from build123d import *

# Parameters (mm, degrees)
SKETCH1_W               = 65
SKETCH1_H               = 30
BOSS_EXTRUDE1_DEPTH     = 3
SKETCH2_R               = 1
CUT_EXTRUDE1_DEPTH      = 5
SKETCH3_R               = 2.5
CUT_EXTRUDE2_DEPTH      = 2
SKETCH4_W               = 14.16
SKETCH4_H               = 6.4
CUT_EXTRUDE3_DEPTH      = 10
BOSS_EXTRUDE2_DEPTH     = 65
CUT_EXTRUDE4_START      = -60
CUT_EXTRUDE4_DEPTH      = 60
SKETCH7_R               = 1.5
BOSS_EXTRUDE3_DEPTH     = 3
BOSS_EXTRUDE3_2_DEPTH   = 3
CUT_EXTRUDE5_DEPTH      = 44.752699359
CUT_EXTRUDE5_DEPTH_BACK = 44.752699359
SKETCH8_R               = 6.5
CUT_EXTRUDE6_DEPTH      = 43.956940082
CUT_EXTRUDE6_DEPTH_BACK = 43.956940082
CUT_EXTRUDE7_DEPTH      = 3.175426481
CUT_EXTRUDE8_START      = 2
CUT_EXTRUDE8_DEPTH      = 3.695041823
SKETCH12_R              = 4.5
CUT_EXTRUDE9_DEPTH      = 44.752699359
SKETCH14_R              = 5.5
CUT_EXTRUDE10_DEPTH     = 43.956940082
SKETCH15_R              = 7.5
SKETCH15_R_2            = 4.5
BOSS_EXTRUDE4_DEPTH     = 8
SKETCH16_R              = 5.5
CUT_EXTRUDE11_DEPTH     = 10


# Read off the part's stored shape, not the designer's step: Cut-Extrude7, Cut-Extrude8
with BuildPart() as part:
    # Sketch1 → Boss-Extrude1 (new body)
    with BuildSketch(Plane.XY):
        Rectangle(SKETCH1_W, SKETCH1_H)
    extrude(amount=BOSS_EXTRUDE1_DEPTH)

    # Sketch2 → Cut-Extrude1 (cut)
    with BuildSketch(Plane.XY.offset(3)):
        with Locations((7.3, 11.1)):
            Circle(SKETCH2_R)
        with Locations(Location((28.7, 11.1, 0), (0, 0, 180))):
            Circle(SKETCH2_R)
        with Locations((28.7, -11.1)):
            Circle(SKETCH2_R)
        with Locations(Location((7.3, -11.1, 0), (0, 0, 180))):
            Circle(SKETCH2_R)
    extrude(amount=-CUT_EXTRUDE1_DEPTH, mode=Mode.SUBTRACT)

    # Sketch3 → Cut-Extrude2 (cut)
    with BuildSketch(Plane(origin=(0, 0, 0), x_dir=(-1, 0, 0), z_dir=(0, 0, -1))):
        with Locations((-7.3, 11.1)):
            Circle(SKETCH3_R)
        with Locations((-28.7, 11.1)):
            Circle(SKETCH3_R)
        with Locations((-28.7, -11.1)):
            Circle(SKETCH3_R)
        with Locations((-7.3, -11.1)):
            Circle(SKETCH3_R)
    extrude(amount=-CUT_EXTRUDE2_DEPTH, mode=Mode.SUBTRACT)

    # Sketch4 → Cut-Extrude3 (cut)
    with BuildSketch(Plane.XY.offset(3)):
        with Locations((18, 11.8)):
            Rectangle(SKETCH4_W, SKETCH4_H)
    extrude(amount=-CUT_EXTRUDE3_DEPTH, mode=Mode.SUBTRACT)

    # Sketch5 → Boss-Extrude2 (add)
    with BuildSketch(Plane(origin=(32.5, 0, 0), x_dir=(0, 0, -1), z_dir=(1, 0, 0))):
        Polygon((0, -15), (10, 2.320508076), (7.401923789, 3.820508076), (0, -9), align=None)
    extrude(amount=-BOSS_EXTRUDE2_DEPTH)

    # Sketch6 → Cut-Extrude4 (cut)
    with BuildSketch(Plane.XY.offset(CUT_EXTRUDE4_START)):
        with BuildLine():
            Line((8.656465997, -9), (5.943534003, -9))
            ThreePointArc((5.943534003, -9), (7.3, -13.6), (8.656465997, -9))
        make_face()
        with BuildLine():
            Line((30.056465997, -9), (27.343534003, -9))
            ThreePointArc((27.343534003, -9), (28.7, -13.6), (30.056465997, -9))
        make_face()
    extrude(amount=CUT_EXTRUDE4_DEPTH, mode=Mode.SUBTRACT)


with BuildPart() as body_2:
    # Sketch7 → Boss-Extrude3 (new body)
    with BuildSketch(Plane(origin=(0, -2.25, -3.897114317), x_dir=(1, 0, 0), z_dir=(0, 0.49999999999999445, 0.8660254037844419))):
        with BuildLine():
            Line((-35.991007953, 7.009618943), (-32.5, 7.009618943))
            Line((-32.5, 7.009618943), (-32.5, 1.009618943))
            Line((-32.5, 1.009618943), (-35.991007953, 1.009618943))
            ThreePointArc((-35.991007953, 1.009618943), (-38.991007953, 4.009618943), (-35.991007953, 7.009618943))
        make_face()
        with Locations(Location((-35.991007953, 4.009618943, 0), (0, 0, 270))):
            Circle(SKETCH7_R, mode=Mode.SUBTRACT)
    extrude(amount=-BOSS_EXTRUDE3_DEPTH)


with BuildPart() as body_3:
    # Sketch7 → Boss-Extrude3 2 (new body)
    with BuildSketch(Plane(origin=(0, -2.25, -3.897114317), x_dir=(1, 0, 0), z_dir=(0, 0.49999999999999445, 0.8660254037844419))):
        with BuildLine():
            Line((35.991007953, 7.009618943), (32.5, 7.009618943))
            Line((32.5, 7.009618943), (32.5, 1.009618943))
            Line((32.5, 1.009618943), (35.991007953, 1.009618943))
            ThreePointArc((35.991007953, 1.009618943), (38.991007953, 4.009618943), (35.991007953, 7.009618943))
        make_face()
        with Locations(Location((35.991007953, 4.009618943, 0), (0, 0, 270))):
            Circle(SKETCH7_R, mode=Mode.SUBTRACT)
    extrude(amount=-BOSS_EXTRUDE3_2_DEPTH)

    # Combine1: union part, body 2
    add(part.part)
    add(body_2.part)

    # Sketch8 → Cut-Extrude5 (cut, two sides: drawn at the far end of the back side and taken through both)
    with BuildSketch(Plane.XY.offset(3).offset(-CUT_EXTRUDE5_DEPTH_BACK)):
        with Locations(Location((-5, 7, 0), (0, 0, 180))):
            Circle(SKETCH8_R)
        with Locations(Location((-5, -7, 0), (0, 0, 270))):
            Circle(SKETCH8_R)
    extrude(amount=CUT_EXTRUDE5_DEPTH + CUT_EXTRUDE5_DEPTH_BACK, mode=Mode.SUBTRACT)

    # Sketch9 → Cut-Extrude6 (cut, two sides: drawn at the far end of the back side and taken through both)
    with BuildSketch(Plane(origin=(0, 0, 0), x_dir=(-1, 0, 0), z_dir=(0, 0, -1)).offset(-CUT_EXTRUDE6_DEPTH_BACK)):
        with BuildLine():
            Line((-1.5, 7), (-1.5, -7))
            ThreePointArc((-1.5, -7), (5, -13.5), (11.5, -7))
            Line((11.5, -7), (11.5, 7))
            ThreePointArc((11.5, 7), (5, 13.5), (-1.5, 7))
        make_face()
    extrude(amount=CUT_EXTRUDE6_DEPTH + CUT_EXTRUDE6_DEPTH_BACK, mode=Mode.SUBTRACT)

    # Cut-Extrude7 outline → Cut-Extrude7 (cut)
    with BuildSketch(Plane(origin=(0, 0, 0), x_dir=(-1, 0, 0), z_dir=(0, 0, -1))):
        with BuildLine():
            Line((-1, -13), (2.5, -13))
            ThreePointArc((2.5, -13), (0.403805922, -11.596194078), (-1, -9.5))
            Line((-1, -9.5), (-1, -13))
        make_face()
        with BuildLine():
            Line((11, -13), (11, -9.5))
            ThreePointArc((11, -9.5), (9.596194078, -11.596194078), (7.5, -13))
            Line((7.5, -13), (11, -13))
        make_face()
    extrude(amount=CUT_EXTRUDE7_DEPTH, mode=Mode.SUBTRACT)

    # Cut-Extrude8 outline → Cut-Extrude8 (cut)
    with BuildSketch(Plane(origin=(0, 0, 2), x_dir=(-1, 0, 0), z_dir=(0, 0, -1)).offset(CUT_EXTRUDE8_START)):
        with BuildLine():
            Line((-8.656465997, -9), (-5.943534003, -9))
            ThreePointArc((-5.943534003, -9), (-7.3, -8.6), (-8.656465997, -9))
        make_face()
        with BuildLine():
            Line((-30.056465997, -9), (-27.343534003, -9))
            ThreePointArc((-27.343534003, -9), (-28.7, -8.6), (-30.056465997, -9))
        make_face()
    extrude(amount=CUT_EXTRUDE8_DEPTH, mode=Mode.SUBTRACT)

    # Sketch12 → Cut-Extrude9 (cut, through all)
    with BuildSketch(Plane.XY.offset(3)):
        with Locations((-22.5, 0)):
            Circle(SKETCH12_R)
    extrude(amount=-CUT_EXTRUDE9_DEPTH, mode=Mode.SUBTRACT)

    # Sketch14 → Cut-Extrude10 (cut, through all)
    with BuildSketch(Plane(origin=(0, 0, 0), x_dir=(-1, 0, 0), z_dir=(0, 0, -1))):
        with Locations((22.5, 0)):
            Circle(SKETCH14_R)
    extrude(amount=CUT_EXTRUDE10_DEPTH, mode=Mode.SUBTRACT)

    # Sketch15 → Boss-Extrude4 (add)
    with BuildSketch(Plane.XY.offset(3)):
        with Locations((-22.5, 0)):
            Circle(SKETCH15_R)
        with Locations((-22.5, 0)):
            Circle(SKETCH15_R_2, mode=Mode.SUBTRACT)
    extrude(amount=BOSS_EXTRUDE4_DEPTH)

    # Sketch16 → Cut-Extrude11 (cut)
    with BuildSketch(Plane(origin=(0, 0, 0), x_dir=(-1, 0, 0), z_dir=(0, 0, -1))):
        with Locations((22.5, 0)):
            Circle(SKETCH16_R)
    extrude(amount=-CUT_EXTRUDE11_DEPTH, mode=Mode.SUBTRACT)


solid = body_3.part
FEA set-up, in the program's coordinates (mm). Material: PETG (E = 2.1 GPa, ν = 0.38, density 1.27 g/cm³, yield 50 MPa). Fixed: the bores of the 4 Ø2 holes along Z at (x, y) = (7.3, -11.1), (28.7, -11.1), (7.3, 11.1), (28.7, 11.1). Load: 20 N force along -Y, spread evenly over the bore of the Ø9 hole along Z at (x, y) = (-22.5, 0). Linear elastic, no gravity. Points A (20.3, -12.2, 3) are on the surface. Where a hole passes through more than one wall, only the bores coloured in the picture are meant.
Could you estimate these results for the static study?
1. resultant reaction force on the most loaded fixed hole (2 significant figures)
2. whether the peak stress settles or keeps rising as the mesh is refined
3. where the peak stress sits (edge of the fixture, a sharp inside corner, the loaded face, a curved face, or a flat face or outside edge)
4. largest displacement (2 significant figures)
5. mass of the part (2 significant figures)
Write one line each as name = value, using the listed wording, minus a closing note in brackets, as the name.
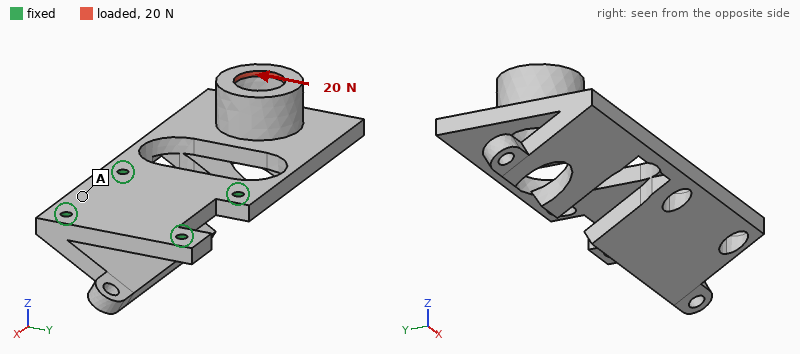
resultant reaction force on the most loaded fixed hole = 23 N
whether the peak stress settles or keeps rising as the mesh is refined = keeps rising
where the peak stress sits = edge of the fixture
largest displacement = 0.85 mm
mass of the part = 9.4 g
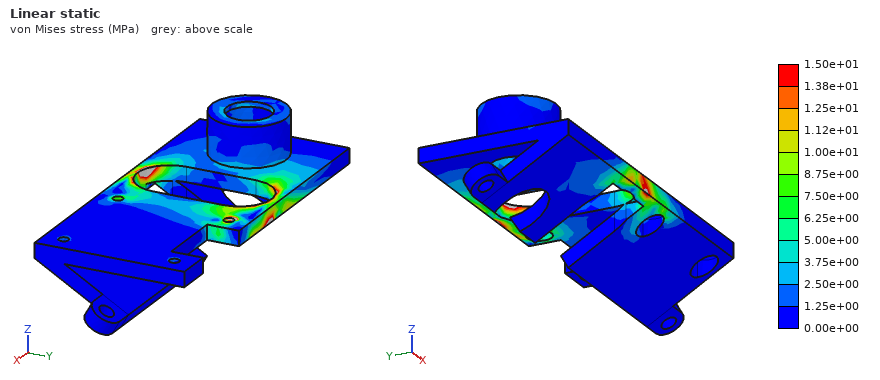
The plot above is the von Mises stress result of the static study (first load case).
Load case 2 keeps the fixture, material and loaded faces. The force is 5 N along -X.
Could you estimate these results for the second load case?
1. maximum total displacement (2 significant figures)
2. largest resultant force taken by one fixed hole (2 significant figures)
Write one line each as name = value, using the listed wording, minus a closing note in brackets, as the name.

maximum total displacement = 1.0 mm
largest resultant force taken by one fixed hole = 4.0 N
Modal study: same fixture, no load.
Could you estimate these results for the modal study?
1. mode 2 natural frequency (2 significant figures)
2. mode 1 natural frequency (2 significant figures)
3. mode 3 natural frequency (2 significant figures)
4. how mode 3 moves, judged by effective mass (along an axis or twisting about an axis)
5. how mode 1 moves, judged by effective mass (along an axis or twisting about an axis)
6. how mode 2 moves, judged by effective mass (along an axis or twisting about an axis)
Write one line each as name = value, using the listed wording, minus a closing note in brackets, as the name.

mode 2 natural frequency = 660 Hz
mode 1 natural frequency = 150 Hz
mode 3 natural frequency = 710 Hz
how mode 3 moves, judged by effective mass = twisting about X
how mode 1 moves, judged by effective mass = along Z
how mode 2 moves, judged by effective mass = along Y
